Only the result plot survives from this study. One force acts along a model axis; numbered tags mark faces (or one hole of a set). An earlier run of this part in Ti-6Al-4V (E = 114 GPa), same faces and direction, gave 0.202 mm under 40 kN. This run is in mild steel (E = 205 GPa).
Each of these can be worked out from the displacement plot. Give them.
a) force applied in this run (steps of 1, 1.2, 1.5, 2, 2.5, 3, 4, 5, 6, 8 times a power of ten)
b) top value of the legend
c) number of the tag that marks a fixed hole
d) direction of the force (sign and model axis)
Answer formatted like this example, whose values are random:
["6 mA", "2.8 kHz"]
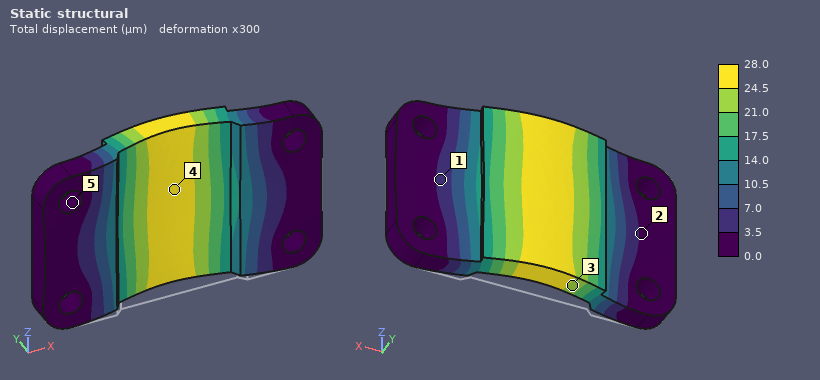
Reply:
["10 kN", "28.0 µm", "5", "+Y"]
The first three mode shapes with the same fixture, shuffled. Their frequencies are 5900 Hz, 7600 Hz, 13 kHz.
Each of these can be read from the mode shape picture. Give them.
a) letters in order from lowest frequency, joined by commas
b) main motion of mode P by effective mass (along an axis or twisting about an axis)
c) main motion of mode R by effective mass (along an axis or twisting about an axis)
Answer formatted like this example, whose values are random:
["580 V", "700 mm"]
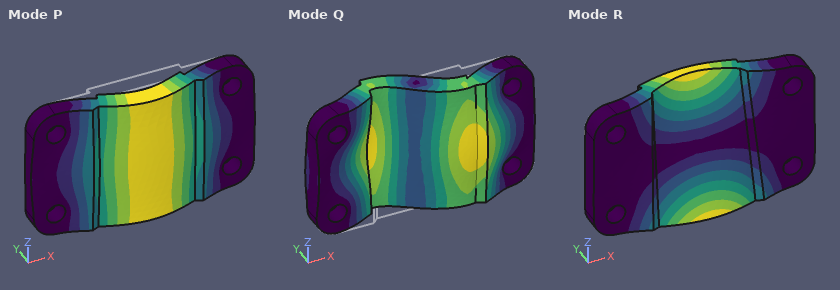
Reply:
["P, R, Q", "along Y", "twisting about X"]
